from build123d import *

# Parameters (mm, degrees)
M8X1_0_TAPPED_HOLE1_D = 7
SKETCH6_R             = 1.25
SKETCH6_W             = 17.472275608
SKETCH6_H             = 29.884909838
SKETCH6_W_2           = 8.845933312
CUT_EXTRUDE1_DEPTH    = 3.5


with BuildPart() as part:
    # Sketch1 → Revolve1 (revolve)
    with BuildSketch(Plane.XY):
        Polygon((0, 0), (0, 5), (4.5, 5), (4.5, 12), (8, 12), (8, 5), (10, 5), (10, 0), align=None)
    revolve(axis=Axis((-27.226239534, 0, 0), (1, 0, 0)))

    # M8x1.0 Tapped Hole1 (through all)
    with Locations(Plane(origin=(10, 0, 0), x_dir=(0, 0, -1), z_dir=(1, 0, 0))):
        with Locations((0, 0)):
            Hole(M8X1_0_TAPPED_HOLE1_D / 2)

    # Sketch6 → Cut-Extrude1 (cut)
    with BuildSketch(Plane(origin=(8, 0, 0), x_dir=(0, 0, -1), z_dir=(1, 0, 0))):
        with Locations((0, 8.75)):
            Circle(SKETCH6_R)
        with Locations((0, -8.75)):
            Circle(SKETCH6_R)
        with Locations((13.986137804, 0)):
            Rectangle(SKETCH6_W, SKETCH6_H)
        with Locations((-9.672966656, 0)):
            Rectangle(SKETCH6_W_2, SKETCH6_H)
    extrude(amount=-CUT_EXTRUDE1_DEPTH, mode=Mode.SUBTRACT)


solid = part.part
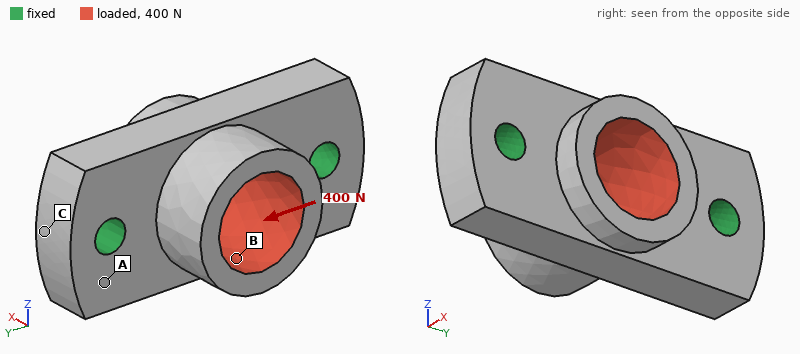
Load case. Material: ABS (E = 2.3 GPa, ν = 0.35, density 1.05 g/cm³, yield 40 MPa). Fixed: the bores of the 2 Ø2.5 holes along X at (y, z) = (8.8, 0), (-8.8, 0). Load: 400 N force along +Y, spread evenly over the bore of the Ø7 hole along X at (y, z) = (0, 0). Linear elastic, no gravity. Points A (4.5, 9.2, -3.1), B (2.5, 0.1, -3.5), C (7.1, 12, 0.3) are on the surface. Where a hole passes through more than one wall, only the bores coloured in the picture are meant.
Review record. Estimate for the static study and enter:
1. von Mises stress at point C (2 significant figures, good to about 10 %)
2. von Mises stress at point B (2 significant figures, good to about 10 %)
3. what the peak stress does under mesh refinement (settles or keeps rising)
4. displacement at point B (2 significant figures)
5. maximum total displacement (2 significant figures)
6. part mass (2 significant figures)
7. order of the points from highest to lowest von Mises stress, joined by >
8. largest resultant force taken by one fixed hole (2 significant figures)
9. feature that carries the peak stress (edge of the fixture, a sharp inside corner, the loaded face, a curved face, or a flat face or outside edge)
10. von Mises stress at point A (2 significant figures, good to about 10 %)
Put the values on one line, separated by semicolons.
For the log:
5.5 MPa; 9.5 MPa; keeps rising; 44 µm; 66 µm; 0.99 g; B > C > A; 200 N; edge of the fixture; 2.7 MPa
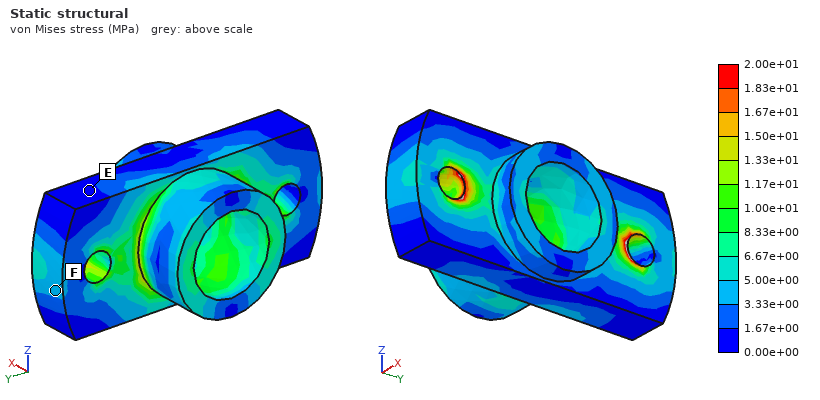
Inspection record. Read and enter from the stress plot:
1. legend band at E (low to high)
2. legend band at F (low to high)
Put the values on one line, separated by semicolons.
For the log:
0.00e+00 to 1.67e+00 MPa; 3.33e+00 to 5.00e+00 MPa
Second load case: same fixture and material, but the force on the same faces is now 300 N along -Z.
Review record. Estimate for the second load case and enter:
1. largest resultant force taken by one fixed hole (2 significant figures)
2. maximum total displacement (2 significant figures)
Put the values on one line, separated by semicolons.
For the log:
150 N; 0.13 mm
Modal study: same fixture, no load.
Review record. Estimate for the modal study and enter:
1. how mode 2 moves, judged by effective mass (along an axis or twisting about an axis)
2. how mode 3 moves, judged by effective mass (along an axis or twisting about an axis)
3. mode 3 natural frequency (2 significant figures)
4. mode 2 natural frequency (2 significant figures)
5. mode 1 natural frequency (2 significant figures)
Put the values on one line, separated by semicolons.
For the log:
along X; along Z; 18 kHz; 13 kHz; 9900 Hz
